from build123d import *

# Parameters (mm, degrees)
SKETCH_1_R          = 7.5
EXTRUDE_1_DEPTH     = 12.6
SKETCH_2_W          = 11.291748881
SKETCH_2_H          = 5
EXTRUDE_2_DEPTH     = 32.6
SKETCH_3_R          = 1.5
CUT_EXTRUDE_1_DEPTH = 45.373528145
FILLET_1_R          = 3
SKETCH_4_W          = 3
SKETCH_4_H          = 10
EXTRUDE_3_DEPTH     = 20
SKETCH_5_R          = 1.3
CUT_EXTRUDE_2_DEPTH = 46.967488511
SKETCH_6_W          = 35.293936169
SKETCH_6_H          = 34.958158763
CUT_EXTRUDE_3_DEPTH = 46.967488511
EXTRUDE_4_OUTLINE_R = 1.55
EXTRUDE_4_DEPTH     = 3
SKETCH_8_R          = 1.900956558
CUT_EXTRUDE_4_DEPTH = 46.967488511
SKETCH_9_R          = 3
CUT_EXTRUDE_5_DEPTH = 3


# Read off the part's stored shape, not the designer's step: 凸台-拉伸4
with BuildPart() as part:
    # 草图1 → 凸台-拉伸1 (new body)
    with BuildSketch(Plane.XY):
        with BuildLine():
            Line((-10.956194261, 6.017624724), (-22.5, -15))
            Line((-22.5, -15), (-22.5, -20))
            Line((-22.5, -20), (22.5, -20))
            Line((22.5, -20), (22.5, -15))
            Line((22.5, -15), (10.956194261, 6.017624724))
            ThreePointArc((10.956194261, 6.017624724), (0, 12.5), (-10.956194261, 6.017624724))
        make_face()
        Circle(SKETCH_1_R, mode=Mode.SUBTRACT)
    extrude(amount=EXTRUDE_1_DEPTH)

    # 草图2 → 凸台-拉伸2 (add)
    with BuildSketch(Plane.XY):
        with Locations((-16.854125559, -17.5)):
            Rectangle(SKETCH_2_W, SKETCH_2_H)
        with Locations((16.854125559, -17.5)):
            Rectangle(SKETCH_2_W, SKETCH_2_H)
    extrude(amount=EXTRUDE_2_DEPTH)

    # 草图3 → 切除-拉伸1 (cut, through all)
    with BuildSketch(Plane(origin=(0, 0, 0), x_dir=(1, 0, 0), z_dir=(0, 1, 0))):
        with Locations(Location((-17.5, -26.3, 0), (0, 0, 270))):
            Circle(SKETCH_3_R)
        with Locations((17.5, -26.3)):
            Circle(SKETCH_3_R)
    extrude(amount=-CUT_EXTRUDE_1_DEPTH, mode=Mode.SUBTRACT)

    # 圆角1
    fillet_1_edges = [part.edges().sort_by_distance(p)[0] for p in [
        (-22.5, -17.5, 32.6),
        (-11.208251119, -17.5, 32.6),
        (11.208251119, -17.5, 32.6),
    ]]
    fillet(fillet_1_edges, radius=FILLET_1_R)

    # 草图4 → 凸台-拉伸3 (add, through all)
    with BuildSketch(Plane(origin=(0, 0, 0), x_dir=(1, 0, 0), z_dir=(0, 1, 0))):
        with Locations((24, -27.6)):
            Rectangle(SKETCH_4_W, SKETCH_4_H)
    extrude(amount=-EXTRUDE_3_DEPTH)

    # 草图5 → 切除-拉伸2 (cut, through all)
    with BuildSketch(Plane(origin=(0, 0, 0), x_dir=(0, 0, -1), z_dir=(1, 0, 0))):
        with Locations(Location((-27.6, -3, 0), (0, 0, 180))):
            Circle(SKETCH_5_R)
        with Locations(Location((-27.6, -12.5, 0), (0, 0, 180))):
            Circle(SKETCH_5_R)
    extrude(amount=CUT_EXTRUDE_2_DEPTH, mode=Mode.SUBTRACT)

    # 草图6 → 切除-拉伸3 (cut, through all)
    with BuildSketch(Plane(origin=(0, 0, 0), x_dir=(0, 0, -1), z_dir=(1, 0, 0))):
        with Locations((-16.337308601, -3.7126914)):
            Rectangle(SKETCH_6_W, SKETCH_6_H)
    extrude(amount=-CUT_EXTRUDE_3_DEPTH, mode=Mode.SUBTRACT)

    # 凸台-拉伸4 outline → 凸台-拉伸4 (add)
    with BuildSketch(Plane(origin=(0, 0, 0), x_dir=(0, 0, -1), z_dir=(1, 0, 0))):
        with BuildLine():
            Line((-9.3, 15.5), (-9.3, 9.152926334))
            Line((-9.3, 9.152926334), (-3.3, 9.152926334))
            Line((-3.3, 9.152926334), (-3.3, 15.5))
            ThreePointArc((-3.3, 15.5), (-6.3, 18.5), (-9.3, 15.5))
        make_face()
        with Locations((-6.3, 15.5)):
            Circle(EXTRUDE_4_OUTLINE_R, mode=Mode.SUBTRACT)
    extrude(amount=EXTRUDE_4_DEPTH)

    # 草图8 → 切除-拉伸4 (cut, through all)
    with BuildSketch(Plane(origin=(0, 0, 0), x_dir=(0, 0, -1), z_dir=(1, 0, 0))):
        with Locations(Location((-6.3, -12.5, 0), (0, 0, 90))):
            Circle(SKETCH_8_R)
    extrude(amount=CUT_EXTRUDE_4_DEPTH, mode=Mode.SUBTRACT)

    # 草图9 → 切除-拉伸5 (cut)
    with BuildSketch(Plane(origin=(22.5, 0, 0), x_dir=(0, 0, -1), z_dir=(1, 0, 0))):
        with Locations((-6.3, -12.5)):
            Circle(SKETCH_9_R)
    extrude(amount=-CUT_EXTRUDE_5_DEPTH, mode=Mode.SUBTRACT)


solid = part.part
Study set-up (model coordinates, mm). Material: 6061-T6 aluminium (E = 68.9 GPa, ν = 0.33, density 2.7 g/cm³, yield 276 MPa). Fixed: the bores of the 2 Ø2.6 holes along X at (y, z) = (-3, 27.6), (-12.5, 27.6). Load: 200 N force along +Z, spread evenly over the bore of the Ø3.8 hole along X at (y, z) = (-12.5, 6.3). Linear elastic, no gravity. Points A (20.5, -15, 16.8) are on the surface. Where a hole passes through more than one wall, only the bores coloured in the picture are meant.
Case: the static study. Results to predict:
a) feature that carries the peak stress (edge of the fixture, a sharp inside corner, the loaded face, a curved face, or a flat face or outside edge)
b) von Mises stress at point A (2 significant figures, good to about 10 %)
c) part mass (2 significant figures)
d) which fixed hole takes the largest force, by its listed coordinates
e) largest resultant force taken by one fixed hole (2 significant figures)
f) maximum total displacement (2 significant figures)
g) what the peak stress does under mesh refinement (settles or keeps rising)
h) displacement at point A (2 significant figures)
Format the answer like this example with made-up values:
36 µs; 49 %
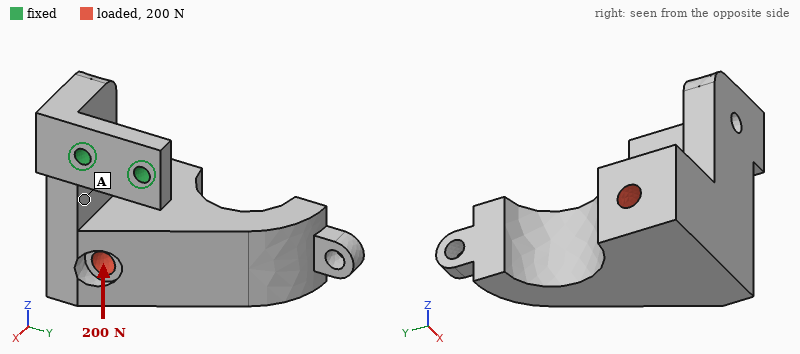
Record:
edge of the fixture; 17 MPa; 18 g; (-12.5, 27.6); 190 N; 0.26 mm; keeps rising; 0.054 mm
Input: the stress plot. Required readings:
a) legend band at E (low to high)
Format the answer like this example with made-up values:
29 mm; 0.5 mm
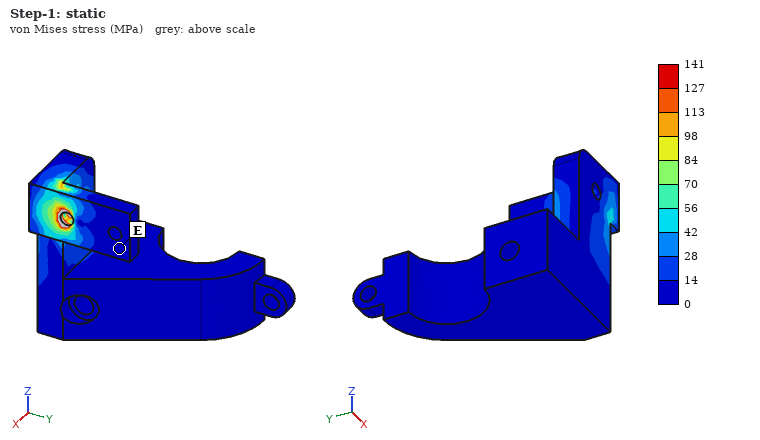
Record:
0 to 14 MPa
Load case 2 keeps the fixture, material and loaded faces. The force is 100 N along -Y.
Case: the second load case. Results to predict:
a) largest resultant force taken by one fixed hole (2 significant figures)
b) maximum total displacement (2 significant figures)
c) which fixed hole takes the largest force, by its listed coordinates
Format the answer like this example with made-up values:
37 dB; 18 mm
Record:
160 N; 0.31 mm; (-12.5, 27.6)
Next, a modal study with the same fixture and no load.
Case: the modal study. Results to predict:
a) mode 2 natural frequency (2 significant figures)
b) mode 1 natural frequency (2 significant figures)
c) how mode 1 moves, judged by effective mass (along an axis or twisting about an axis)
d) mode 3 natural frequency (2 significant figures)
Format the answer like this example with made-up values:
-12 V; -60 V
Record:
1100 Hz; 930 Hz; along Y; 2400 Hz
